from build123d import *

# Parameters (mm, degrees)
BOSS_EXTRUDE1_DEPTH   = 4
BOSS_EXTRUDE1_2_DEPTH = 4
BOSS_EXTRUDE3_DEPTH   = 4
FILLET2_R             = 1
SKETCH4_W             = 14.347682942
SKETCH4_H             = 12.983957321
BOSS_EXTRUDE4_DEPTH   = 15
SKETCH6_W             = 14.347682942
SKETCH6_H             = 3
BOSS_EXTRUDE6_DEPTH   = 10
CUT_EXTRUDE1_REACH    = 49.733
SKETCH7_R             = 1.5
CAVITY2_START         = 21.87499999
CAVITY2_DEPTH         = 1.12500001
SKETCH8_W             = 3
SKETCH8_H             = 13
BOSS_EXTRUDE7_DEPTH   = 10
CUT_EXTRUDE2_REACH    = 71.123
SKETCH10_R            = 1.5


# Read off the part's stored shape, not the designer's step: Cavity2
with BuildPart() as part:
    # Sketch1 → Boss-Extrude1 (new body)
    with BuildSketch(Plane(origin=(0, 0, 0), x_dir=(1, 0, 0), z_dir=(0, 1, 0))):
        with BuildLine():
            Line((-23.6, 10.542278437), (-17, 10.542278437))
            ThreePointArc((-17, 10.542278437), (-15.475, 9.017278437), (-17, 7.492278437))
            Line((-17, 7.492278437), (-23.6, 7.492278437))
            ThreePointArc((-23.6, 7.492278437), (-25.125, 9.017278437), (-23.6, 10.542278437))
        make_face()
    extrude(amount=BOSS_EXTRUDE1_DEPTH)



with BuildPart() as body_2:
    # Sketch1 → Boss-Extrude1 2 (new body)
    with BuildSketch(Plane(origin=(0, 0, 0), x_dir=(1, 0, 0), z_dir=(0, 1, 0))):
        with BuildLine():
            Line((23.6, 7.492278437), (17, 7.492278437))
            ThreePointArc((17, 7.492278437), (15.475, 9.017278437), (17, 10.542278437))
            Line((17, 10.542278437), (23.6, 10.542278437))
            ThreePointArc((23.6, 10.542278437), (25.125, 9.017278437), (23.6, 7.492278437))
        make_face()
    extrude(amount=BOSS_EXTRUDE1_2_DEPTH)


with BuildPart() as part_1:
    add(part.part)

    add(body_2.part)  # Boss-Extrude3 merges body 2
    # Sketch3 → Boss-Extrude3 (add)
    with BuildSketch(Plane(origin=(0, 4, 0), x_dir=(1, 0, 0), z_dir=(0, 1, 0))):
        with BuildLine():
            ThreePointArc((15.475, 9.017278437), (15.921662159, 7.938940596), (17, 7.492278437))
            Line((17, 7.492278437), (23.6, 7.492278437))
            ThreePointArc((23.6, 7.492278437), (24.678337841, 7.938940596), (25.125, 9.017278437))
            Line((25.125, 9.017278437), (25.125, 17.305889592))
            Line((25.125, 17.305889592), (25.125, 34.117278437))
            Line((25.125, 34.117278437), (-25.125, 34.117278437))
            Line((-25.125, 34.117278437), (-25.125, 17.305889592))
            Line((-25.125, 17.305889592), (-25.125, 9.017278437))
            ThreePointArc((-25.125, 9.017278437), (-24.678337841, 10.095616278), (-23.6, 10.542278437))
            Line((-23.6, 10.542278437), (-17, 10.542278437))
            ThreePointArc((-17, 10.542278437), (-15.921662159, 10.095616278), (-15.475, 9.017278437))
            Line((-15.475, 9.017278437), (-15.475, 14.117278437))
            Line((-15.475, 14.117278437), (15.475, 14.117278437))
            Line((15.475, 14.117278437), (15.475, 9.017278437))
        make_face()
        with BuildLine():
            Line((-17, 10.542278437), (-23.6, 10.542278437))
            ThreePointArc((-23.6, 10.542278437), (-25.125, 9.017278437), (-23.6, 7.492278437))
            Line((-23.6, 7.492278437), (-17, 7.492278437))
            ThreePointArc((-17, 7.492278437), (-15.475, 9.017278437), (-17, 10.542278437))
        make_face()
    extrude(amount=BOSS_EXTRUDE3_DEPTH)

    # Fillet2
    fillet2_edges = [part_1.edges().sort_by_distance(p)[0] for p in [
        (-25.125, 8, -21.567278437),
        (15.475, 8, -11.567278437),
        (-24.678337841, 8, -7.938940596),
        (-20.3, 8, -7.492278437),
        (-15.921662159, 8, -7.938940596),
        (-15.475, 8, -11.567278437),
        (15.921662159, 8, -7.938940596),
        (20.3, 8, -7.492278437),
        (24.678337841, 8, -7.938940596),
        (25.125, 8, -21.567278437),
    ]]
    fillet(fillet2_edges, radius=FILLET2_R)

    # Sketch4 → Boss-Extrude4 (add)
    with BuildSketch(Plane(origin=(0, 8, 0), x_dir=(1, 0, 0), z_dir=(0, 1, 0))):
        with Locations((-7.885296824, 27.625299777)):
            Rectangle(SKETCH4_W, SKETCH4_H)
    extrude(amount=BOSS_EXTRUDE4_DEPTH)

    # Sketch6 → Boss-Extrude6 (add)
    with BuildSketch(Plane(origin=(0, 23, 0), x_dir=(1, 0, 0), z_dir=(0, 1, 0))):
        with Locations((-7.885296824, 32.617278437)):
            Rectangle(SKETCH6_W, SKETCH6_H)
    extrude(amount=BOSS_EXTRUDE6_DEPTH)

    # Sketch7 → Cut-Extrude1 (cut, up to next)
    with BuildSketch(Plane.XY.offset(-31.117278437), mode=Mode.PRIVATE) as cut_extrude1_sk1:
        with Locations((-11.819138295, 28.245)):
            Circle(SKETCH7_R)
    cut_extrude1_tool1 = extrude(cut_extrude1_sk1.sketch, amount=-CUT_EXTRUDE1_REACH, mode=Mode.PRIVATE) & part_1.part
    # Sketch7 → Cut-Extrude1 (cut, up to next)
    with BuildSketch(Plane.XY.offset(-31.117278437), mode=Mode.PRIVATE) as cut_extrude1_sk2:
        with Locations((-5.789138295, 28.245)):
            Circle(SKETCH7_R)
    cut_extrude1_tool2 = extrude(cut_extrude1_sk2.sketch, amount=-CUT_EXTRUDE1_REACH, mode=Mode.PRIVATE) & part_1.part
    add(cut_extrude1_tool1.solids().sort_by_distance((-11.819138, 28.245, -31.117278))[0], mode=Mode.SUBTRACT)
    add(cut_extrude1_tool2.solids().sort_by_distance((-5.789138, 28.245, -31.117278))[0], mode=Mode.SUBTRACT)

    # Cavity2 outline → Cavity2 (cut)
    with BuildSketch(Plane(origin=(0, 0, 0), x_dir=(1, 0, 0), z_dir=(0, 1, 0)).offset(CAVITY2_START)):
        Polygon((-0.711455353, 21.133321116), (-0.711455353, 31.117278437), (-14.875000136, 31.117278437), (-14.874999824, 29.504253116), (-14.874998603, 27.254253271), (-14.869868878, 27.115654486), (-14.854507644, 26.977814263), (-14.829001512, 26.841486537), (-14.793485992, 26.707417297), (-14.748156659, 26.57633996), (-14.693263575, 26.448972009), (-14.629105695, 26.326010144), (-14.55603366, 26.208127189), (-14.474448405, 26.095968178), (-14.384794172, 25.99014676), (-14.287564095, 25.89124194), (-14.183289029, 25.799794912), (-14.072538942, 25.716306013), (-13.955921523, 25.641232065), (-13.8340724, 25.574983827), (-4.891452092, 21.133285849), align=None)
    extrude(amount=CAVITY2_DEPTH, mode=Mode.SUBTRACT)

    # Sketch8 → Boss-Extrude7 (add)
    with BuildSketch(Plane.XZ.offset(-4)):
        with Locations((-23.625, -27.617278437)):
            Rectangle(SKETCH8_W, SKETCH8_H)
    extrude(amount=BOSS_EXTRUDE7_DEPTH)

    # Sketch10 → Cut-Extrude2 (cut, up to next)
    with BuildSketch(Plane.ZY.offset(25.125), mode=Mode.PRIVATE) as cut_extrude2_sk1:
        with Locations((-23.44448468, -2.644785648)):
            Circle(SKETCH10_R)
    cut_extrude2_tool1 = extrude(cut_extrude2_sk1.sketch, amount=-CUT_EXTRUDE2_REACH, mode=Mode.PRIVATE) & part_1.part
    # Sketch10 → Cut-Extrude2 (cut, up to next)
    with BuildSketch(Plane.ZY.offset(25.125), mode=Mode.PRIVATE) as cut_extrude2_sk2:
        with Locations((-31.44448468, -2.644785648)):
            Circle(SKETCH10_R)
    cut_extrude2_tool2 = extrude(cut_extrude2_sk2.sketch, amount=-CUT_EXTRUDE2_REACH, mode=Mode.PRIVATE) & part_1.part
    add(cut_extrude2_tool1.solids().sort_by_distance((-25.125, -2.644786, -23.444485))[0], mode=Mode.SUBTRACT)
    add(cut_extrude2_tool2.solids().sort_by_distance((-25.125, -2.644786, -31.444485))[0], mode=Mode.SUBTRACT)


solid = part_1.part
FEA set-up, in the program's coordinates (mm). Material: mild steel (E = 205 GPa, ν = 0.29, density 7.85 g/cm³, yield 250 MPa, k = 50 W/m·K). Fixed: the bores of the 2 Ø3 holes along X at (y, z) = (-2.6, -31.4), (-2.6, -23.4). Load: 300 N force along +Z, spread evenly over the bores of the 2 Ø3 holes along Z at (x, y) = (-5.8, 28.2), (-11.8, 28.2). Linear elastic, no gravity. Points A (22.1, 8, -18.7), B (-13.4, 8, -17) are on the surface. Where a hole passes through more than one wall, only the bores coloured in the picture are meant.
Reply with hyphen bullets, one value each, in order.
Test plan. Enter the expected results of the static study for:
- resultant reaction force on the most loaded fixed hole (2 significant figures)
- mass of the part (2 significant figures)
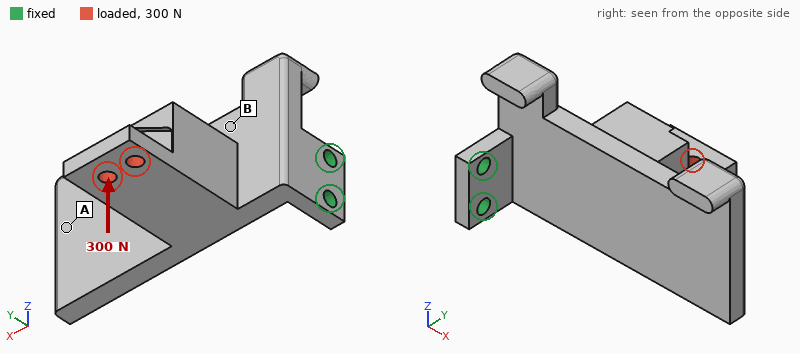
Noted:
- 1.1 kN
- 64 g
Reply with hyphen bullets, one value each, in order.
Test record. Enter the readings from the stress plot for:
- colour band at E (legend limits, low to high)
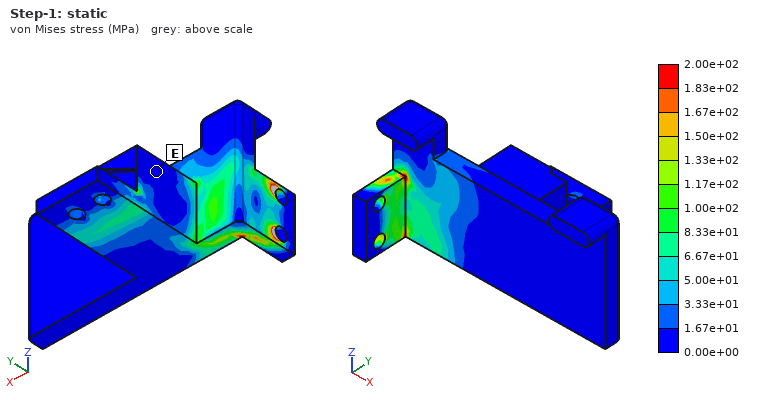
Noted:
- 0.00e+00 to 1.67e+01 MPa
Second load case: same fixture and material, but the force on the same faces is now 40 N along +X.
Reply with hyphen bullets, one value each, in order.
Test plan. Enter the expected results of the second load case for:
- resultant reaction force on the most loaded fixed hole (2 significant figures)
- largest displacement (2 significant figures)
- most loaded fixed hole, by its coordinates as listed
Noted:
- 42 N
- 79 µm
- (-2.6, -31.4)
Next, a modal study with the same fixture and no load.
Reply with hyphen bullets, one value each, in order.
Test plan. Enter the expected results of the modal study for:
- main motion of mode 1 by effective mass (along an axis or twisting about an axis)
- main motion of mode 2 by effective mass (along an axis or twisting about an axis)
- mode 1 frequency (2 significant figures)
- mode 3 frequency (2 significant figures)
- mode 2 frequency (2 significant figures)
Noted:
- along Y
- along Z
- 630 Hz
- 3200 Hz
- 1300 Hz
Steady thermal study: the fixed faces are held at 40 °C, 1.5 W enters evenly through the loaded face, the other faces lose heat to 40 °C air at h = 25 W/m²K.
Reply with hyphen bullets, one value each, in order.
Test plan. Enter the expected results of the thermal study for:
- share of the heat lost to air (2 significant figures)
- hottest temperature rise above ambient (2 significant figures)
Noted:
- 44 %
- 15 K
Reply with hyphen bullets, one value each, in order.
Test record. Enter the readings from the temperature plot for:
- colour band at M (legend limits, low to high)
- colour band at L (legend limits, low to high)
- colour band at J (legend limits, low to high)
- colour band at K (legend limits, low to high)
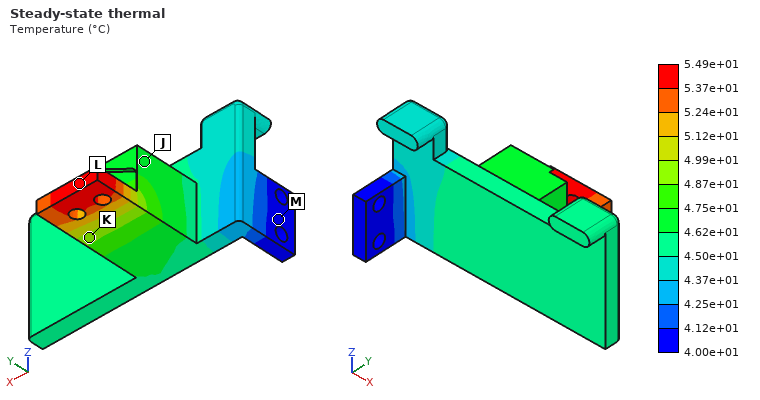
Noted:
- 4.00e+01 to 4.12e+01 °C
- 5.37e+01 to 5.49e+01 °C
- 4.62e+01 to 4.75e+01 °C
- 4.87e+01 to 4.99e+01 °C
